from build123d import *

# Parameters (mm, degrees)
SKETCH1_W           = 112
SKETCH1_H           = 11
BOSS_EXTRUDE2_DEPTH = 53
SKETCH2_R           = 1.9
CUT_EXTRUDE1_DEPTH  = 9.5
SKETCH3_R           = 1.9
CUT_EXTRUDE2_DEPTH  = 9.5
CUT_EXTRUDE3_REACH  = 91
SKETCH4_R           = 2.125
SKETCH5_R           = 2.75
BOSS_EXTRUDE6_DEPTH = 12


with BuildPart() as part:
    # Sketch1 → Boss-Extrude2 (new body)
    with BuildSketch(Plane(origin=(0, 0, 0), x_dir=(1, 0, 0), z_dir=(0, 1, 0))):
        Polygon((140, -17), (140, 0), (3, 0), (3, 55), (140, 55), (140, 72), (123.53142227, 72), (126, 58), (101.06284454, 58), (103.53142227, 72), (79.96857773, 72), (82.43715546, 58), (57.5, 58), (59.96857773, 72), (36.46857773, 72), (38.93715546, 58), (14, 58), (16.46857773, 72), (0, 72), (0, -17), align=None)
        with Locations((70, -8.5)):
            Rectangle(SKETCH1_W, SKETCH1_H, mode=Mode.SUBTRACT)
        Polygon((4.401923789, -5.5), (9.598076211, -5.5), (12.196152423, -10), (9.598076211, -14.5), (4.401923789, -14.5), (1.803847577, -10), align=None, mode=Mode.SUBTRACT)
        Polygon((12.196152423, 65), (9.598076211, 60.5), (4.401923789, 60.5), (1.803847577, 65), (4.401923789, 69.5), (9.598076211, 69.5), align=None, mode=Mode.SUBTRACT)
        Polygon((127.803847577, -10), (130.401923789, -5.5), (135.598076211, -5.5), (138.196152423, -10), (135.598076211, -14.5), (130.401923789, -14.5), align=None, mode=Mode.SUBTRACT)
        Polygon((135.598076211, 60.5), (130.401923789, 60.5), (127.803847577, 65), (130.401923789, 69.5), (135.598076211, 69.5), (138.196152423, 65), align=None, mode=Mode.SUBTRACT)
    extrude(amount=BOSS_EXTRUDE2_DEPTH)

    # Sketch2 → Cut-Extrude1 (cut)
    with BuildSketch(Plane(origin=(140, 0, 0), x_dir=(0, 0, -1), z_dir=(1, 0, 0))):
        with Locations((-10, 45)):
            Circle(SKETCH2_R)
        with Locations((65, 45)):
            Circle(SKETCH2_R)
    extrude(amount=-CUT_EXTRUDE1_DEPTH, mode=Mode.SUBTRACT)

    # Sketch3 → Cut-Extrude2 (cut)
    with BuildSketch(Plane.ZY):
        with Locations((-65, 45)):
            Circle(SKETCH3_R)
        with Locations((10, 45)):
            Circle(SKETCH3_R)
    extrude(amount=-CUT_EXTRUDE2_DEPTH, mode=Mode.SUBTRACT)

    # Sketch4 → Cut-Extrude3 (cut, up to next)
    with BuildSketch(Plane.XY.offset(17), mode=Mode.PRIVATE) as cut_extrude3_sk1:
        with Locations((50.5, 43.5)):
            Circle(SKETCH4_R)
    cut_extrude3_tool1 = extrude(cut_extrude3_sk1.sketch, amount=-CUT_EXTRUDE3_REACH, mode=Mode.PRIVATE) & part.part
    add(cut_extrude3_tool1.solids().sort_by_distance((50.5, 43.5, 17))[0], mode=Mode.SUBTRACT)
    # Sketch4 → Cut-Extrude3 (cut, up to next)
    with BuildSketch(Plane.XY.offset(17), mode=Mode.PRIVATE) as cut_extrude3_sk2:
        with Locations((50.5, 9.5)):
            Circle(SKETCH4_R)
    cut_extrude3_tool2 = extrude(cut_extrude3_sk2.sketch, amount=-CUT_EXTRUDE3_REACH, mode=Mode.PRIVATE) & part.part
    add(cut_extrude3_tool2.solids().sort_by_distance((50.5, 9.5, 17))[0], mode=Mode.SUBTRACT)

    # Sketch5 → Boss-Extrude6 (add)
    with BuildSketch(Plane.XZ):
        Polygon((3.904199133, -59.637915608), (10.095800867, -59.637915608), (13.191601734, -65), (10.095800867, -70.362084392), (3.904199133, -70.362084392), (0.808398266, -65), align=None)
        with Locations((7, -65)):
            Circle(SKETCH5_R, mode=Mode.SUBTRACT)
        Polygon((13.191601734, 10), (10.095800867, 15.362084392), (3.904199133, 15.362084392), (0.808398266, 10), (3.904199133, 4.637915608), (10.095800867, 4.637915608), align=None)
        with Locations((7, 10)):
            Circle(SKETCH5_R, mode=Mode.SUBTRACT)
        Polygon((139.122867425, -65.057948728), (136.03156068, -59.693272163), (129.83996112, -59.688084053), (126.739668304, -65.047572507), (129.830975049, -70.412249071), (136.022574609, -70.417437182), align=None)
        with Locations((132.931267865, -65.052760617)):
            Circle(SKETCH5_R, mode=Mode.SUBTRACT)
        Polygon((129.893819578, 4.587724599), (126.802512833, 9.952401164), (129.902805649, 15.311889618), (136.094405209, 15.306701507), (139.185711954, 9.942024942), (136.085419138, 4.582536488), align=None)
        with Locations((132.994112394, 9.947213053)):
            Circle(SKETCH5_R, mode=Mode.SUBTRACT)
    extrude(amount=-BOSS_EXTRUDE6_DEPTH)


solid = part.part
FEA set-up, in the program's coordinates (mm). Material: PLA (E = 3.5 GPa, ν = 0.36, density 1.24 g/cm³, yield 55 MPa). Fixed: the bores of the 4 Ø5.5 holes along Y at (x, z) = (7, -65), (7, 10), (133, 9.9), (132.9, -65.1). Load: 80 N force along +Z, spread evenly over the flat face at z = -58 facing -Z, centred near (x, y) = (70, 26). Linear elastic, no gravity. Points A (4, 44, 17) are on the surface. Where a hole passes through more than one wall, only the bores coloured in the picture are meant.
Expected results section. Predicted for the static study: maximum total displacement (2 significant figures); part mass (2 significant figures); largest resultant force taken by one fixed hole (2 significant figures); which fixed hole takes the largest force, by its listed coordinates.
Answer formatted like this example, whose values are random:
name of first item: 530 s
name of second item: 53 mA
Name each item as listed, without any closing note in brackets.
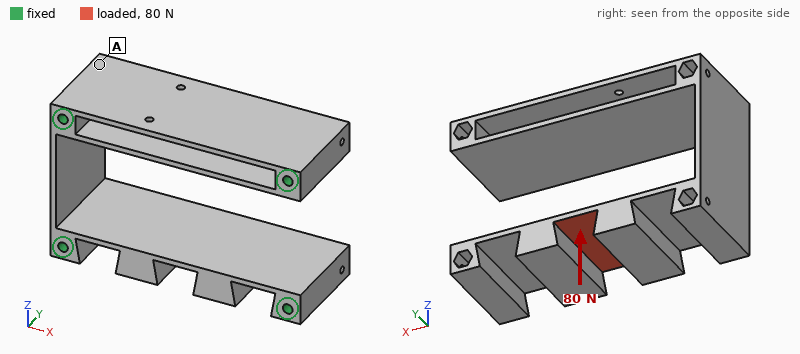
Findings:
maximum total displacement: 1.3 mm
part mass: 160 g
largest resultant force taken by one fixed hole: 57 N
which fixed hole takes the largest force, by its listed coordinates: (7, -65)
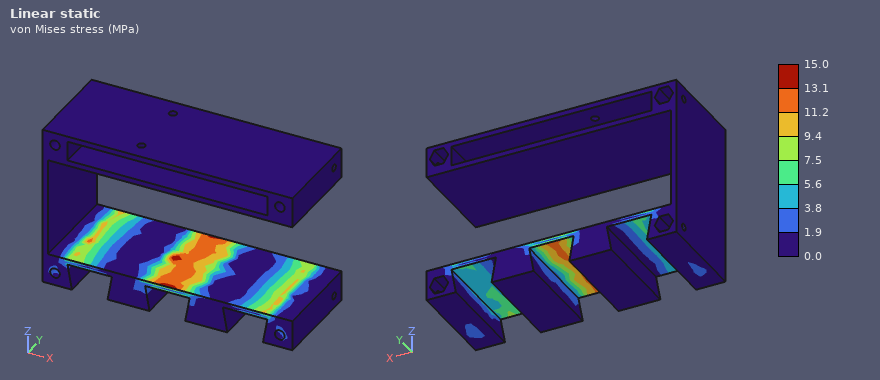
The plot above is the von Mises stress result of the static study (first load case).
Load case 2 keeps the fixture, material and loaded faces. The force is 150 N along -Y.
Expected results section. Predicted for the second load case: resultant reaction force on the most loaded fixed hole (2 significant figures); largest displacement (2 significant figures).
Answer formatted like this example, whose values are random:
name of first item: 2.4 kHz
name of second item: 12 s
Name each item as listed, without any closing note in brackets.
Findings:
resultant reaction force on the most loaded fixed hole: 89 N
largest displacement: 73 µm
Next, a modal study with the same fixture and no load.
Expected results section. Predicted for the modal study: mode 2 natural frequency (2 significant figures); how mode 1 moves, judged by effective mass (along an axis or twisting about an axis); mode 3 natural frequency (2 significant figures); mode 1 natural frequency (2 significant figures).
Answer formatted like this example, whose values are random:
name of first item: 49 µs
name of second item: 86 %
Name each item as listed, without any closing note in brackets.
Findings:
mode 2 natural frequency: 390 Hz
how mode 1 moves, judged by effective mass: along Z
mode 3 natural frequency: 400 Hz
mode 1 natural frequency: 240 Hz
